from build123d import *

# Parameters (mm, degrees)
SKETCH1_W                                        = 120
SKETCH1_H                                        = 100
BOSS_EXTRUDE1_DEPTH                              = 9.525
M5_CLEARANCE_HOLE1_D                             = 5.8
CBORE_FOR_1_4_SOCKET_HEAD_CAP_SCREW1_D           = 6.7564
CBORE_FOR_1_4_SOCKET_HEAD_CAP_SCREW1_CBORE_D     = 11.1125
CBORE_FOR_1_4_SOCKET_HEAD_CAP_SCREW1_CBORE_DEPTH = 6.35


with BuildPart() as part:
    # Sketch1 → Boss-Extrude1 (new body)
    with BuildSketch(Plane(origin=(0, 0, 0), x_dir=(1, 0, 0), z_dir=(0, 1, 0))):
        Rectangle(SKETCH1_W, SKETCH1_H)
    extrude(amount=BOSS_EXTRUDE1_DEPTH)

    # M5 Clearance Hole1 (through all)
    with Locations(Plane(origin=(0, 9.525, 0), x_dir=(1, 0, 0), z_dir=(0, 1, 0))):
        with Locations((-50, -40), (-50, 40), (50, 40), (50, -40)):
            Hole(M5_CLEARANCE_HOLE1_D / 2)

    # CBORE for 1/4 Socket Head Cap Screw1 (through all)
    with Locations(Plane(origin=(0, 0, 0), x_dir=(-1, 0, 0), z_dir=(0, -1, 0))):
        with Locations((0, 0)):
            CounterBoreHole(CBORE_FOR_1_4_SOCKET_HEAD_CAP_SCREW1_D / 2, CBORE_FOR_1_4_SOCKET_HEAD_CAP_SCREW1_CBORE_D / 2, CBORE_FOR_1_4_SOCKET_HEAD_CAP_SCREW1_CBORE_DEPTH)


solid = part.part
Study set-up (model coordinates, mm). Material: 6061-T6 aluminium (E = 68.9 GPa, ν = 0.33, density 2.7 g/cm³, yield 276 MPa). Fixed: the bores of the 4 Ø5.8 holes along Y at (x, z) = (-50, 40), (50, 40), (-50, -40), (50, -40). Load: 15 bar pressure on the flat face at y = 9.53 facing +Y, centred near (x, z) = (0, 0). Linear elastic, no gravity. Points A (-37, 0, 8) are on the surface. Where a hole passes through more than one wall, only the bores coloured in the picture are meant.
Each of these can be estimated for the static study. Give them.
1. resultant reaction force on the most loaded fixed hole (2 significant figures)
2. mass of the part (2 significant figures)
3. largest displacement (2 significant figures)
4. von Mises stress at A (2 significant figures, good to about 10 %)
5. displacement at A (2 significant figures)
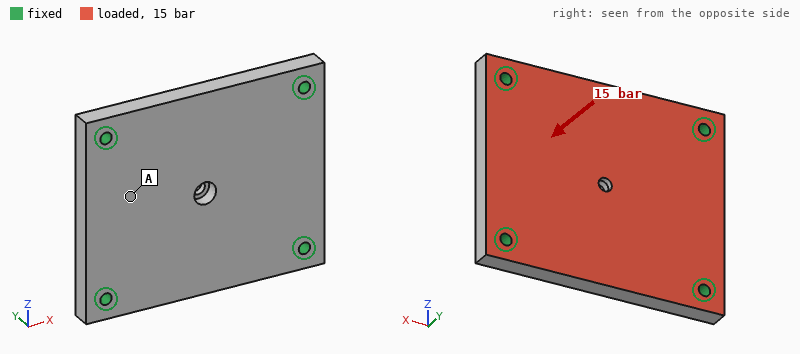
4.5 kN
300 g
0.17 mm
32 MPa
0.091 mm
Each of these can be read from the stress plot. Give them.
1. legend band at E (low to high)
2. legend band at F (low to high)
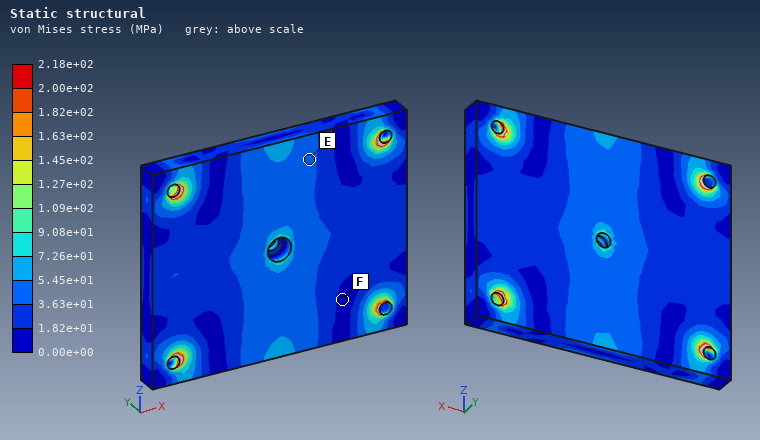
3.63e+01 to 5.45e+01 MPa
0.00e+00 to 1.82e+01 MPa
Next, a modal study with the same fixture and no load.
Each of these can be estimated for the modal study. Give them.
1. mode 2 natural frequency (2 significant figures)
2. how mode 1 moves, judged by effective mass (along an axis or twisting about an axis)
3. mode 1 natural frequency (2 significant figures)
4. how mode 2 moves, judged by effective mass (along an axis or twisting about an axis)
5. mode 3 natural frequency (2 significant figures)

5400 Hz
along Y
3600 Hz
twisting about X
6800 Hz
